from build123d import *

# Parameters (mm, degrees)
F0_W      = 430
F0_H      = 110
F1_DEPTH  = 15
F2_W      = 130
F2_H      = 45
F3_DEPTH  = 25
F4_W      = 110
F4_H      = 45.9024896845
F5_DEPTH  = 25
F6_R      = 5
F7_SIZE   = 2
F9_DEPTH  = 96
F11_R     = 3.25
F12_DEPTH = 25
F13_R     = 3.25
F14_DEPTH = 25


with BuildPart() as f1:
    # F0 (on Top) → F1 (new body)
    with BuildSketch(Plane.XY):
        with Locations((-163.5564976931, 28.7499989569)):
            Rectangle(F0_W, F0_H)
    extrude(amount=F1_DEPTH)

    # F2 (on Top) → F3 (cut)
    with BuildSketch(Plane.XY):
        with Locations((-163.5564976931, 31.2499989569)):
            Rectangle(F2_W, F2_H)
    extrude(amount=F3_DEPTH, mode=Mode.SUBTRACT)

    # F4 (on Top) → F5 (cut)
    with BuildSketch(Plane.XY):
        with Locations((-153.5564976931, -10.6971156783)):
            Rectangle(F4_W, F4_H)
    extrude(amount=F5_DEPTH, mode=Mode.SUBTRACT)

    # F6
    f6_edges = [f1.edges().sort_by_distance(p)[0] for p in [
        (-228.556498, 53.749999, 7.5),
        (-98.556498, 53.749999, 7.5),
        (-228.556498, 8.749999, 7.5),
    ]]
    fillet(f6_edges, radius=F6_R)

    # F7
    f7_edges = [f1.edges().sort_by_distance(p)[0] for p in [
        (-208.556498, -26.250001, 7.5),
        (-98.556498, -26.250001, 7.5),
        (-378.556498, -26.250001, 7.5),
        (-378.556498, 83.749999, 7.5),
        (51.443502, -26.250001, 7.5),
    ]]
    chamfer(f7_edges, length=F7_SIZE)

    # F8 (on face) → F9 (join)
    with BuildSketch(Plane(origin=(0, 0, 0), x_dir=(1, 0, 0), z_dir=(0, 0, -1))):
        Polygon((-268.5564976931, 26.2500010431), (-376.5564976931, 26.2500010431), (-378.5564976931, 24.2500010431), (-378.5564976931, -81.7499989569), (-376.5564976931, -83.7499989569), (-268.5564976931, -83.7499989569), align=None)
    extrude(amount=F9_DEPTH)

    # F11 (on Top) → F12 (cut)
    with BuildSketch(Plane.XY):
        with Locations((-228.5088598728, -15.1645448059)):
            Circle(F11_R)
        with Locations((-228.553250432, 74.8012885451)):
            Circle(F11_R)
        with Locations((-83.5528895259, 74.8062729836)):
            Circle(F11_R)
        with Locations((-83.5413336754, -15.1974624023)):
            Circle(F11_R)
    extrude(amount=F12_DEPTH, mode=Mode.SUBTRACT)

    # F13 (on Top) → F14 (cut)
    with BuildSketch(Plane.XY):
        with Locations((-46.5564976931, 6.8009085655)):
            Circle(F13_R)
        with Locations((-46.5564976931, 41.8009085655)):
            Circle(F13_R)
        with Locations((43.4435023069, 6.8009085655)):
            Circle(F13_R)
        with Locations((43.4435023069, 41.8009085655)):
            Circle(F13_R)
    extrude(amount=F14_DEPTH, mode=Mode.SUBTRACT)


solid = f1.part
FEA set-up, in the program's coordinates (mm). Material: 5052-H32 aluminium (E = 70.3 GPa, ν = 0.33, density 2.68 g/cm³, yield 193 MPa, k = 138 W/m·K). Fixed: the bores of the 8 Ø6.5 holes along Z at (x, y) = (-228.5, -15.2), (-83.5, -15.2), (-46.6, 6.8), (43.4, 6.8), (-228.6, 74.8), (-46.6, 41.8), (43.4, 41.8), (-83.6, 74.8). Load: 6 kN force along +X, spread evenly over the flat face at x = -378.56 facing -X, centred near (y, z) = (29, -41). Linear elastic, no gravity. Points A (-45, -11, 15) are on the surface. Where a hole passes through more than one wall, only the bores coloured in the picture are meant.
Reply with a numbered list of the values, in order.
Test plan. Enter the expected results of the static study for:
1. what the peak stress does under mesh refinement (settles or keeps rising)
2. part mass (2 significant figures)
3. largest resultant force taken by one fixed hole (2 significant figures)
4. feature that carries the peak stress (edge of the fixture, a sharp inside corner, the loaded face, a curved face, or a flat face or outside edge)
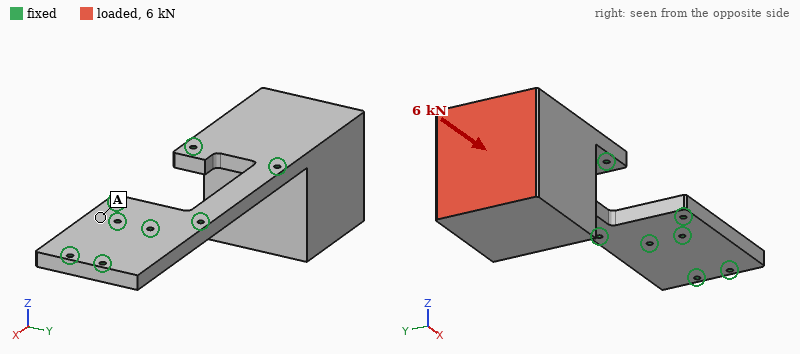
1. keeps rising
2. 4.6 kg
3. 3.2 kN
4. edge of the fixture
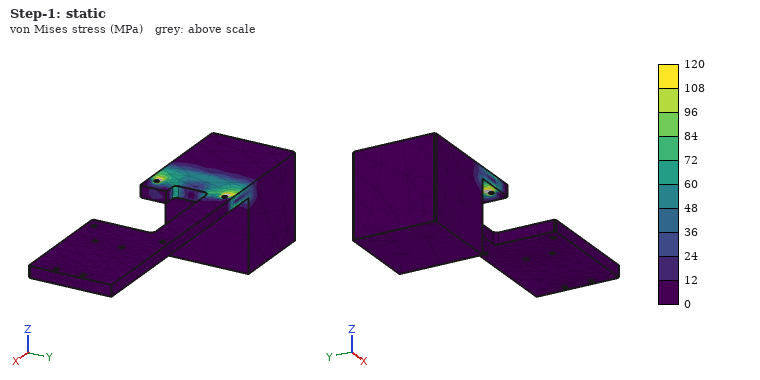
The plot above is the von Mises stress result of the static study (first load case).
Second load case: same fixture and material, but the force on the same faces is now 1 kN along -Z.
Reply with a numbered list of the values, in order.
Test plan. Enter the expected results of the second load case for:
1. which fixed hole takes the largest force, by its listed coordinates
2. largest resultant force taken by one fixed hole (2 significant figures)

1. (-228.6, 74.8)
2. 600 N
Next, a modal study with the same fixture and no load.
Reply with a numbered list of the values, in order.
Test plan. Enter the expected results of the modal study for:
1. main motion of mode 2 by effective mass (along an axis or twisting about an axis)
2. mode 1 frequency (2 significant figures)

1. along Y
2. 160 Hz
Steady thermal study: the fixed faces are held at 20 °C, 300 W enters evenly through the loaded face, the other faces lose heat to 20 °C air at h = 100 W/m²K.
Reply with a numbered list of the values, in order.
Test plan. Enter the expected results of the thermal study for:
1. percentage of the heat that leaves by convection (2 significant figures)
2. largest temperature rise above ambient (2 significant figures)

1. 72 %
2. 44 K
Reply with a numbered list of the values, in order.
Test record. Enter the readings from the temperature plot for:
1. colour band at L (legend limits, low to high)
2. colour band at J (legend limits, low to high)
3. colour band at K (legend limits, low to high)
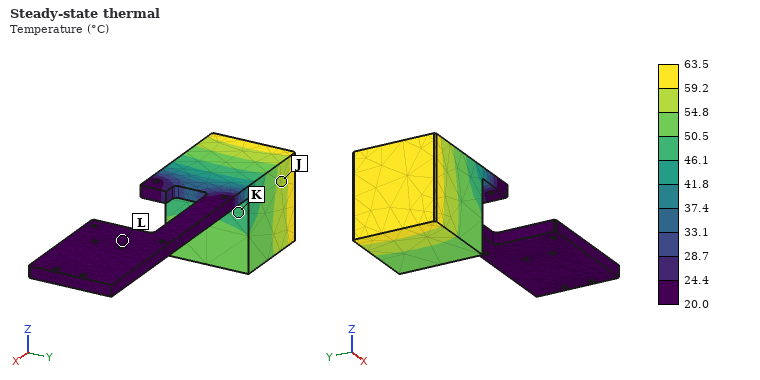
1. 20.0 to 24.4 °C
2. 54.8 to 59.2 °C
3. 46.1 to 50.5 °C
